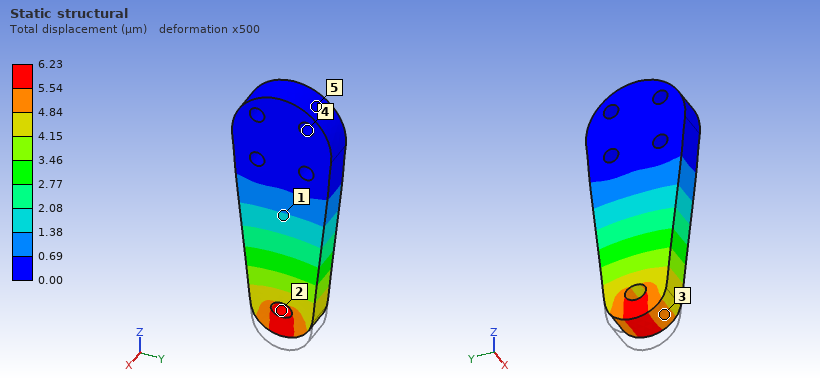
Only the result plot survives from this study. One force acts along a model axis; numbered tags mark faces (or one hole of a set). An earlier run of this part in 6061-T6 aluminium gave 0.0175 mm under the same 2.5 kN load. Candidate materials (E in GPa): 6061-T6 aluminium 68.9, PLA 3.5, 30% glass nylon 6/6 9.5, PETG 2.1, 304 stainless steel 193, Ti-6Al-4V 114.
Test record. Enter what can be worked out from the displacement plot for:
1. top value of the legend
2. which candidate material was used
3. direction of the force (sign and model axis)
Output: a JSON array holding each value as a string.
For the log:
["6.23 µm", "304 stainless steel", "+Z"]
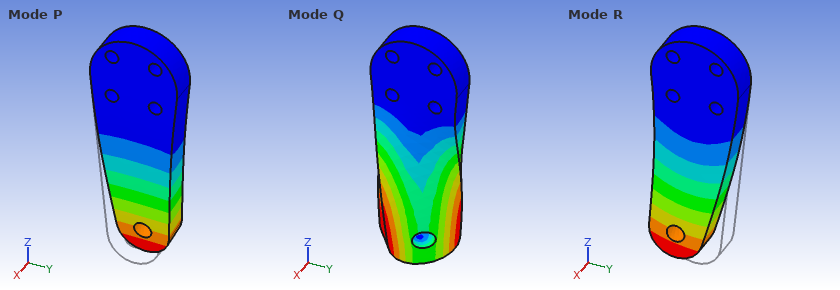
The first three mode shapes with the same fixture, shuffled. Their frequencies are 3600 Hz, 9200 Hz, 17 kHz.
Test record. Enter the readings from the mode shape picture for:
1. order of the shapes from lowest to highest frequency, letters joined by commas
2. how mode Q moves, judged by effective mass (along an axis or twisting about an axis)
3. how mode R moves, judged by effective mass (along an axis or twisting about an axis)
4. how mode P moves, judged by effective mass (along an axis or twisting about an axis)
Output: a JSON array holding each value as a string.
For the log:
["P, R, Q", "twisting about Z", "along Y", "along X"]
